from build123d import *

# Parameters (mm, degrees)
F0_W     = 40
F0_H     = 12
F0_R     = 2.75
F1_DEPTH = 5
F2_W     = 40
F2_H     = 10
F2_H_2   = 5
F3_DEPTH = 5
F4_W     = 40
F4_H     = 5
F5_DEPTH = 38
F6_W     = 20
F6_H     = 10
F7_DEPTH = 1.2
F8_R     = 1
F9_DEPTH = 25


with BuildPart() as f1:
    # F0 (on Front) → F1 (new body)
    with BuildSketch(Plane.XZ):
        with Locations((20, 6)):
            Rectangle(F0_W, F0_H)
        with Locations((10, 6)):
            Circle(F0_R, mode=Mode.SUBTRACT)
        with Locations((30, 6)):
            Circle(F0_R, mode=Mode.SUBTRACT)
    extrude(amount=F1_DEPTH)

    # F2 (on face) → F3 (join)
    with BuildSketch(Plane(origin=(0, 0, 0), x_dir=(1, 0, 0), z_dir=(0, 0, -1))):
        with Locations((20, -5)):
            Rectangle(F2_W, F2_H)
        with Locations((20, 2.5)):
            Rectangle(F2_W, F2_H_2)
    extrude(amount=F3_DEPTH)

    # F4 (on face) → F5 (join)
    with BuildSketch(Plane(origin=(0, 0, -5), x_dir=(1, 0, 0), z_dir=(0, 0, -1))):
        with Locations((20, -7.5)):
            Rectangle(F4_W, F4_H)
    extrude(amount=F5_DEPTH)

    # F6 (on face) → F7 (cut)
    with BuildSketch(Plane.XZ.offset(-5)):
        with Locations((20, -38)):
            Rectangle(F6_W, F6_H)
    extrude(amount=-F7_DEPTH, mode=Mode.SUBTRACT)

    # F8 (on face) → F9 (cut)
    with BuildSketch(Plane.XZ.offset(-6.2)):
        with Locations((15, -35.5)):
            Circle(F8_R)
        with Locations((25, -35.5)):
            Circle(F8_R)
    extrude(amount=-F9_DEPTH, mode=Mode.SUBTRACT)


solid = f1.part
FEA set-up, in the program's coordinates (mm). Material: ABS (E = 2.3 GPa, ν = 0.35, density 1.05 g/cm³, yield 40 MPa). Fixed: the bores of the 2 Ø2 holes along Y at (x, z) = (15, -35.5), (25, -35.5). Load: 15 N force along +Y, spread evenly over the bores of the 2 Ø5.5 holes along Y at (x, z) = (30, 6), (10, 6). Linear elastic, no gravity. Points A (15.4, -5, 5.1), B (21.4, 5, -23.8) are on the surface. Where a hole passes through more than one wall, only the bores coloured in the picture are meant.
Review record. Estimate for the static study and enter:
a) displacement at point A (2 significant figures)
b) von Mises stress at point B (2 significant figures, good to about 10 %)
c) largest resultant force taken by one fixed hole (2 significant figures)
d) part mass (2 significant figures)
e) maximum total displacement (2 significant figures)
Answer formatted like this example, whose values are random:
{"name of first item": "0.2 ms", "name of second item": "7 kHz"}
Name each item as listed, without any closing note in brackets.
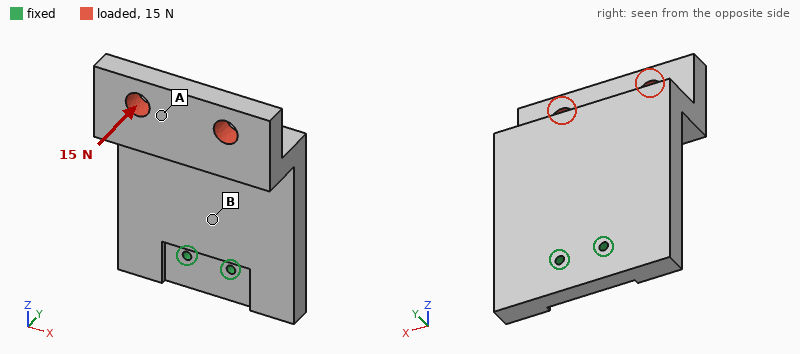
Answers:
{"displacement at point A": "0.66 mm", "von Mises stress at point B": "2.5 MPa", "largest resultant force taken by one fixed hole": "7.6 N", "part mass": "13 g", "maximum total displacement": "0.80 mm"}
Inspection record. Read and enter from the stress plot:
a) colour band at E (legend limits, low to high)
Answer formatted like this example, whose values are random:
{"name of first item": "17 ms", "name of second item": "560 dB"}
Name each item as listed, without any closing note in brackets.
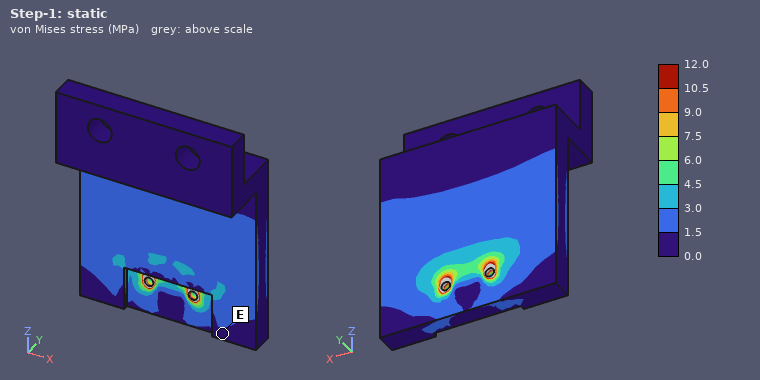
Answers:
{"colour band at E": "0.0 to 1.5 MPa"}
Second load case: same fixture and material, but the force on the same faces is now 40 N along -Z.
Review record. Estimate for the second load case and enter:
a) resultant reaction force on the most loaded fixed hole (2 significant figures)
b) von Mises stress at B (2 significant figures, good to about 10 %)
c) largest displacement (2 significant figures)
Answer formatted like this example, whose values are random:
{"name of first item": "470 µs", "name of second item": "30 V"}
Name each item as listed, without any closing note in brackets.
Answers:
{"resultant reaction force on the most loaded fixed hole": "20 N", "von Mises stress at B": "2.5 MPa", "largest displacement": "0.69 mm"}
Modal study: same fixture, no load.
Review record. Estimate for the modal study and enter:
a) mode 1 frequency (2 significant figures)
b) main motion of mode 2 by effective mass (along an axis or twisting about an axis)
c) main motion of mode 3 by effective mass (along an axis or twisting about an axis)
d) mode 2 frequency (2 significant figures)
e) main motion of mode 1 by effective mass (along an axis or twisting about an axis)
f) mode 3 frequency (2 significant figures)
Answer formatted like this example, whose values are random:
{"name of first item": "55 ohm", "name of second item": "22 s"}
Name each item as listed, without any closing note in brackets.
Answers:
{"mode 1 frequency": "340 Hz", "main motion of mode 2 by effective mass": "along X", "main motion of mode 3 by effective mass": "along X", "mode 2 frequency": "820 Hz", "main motion of mode 1 by effective mass": "along Y", "mode 3 frequency": "1200 Hz"}
